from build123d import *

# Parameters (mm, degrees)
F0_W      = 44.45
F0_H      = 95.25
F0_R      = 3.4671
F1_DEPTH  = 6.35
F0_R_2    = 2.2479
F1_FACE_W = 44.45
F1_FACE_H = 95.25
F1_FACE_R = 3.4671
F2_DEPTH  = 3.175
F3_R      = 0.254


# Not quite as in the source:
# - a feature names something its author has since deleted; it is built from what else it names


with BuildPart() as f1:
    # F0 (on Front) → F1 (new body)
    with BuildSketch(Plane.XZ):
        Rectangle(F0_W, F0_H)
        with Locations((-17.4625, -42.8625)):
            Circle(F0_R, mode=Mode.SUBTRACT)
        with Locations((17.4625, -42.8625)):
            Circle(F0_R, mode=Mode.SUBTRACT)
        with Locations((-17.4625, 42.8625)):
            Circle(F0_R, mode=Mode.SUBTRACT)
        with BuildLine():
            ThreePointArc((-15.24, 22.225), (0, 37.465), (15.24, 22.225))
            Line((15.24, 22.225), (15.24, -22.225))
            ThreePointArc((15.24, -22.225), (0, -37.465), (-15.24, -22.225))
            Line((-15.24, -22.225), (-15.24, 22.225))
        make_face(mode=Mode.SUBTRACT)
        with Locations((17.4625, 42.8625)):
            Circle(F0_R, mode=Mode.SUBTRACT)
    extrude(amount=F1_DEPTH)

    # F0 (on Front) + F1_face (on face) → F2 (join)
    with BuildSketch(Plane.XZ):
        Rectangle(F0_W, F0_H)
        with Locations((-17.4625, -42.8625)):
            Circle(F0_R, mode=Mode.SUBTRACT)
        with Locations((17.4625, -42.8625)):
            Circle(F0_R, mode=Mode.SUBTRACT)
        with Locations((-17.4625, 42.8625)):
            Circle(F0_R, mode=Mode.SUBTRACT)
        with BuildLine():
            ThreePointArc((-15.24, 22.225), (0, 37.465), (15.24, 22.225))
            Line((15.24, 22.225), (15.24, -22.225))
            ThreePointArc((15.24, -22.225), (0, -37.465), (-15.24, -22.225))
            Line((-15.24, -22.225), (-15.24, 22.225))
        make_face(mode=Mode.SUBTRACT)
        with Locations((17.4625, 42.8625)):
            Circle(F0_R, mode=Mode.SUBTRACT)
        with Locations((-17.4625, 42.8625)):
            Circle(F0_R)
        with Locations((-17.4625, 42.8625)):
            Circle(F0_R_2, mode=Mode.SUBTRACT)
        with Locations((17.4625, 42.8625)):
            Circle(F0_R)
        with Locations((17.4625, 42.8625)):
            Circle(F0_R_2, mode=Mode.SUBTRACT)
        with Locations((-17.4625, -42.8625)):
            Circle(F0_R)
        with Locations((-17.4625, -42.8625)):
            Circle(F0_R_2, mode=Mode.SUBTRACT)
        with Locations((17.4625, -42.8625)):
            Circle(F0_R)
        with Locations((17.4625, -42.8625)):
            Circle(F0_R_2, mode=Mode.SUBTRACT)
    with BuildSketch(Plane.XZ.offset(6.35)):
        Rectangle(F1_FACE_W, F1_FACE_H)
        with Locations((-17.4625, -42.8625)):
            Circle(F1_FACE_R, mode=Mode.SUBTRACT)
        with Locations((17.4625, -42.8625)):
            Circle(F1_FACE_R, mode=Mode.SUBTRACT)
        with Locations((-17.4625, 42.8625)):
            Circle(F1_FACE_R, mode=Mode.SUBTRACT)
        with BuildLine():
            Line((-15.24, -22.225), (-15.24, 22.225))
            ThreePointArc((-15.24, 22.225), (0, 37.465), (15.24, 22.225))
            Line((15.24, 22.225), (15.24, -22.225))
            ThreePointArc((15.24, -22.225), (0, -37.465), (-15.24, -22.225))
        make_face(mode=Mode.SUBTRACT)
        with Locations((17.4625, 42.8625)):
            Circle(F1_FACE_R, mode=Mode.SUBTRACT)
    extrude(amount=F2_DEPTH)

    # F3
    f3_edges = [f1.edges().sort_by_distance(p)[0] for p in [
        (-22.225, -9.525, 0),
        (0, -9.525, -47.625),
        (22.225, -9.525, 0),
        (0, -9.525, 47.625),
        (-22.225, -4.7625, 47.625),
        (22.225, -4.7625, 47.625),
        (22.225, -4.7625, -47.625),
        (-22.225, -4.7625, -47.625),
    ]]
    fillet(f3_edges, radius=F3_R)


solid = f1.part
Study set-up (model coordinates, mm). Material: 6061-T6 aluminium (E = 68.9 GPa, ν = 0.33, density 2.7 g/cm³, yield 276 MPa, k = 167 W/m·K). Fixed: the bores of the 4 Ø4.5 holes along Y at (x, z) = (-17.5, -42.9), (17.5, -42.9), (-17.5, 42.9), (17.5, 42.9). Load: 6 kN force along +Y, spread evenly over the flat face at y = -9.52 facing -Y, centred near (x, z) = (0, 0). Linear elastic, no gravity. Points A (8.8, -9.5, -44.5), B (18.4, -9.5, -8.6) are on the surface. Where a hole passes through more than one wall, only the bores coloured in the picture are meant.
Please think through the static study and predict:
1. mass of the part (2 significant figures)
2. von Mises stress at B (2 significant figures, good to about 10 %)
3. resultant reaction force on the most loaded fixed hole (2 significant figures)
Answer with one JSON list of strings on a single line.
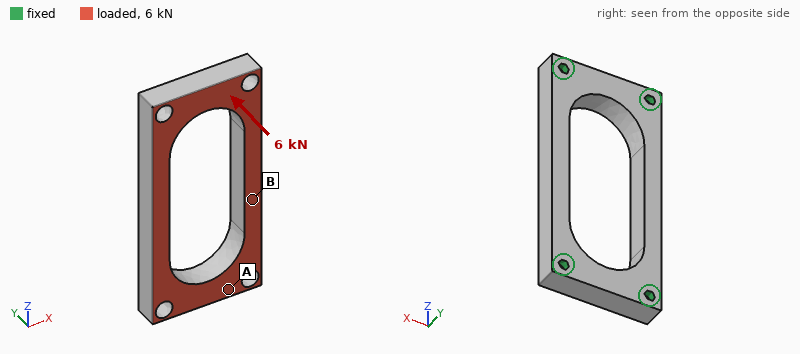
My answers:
["52 g", "83 MPa", "1.9 kN"]
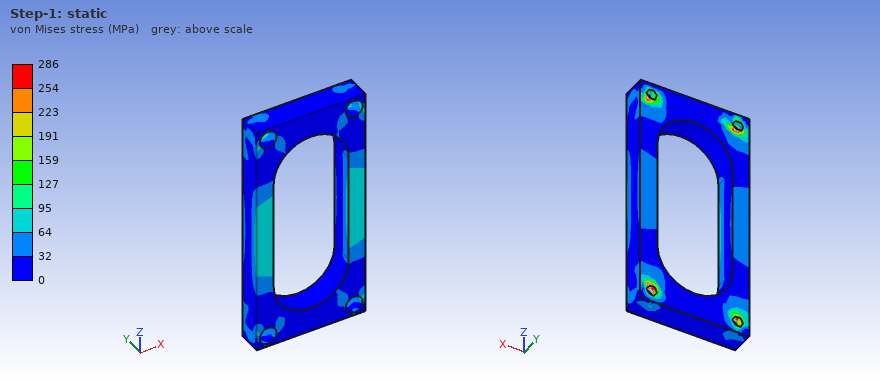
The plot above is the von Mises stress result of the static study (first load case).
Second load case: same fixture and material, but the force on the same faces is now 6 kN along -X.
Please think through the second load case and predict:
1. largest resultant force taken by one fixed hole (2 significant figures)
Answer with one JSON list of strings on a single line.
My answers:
["1.6 kN"]
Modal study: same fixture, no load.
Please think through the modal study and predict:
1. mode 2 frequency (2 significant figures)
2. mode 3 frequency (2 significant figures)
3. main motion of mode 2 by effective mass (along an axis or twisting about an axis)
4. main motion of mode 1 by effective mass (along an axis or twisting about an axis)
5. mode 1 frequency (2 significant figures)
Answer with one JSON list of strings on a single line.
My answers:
["6000 Hz", "6400 Hz", "twisting about Z", "along Y", "5300 Hz"]
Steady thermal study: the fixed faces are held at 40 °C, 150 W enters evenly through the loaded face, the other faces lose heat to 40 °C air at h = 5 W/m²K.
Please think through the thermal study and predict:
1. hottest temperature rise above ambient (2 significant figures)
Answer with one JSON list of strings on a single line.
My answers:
["47 K"]
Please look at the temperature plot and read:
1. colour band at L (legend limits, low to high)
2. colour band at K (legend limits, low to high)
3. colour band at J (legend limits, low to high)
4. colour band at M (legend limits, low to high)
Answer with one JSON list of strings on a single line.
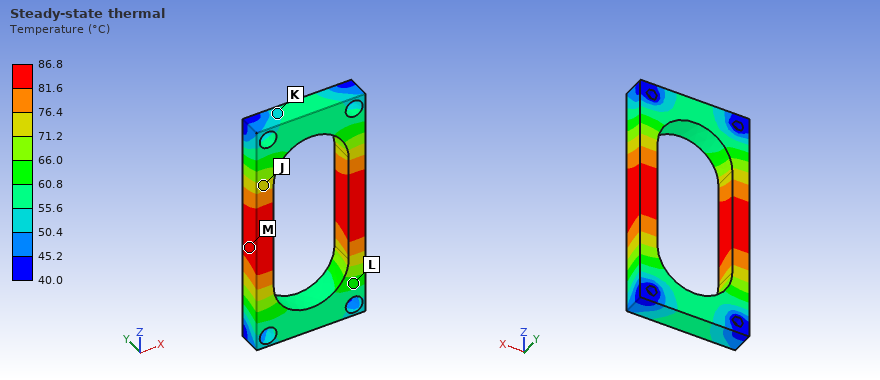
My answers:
["60.8 to 66.0 °C", "50.4 to 55.6 °C", "71.2 to 76.4 °C", "81.6 to 86.8 °C"]
